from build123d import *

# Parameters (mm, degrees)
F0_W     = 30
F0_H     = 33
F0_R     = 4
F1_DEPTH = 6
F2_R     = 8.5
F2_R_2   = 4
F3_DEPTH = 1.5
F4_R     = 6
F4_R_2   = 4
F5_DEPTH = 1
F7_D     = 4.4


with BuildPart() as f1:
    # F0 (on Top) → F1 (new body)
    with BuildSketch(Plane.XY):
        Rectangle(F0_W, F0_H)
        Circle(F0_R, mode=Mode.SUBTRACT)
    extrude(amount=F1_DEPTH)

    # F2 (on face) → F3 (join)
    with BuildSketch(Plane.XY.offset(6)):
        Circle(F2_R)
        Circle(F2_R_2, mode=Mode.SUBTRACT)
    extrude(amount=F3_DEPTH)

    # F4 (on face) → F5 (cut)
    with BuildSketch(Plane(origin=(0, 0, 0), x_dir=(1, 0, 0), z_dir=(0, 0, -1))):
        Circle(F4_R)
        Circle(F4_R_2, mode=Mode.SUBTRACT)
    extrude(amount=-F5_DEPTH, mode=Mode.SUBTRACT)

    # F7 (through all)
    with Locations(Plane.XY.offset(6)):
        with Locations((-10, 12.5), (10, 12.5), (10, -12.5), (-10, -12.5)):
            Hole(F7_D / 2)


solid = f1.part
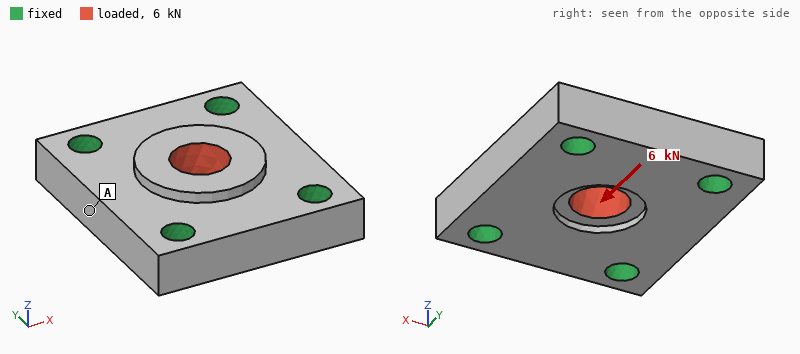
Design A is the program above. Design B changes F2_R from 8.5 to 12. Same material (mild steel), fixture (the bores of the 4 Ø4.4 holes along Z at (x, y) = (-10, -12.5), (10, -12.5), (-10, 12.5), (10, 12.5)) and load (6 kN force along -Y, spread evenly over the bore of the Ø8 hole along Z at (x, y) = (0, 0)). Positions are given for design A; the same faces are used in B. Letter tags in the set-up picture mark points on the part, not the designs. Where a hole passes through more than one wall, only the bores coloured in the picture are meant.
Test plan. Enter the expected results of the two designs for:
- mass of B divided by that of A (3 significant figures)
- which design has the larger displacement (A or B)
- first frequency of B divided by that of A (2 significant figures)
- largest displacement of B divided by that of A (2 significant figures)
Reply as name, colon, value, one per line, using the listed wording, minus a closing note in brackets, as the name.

mass of B divided by that of A: 1.06
which design has the larger displacement: A
first frequency of B divided by that of A: 1.00
largest displacement of B divided by that of A: 0.86
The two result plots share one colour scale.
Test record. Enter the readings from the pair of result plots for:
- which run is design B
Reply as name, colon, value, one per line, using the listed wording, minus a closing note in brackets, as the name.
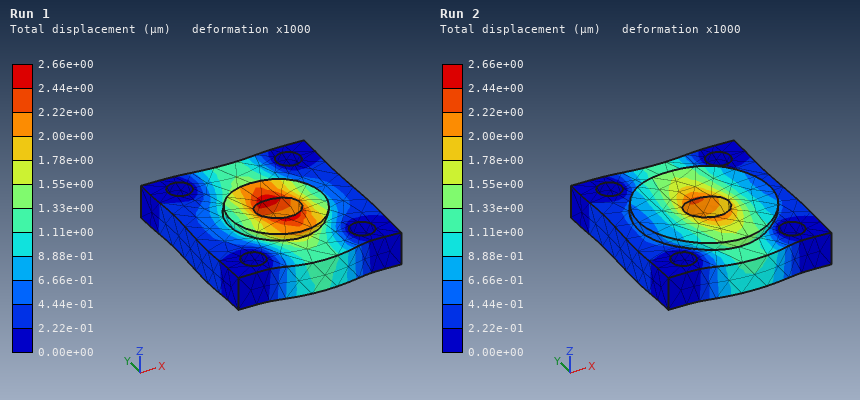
which run is design B: Run 2
